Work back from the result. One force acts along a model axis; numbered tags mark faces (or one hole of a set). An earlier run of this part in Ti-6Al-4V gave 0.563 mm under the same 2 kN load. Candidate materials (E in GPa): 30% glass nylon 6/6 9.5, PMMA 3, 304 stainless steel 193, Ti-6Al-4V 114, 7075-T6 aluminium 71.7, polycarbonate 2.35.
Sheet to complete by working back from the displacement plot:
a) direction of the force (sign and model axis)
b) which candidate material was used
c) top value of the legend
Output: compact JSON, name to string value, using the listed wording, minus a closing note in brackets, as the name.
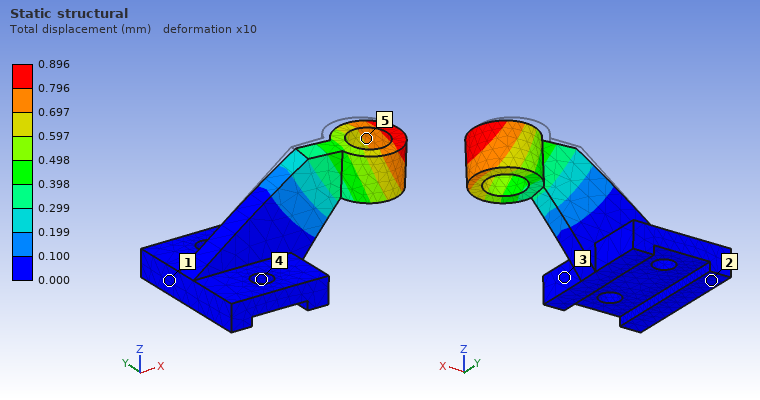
{"direction of the force": "-Y", "which candidate material was used": "7075-T6 aluminium", "top value of the legend": "0.896 mm"}
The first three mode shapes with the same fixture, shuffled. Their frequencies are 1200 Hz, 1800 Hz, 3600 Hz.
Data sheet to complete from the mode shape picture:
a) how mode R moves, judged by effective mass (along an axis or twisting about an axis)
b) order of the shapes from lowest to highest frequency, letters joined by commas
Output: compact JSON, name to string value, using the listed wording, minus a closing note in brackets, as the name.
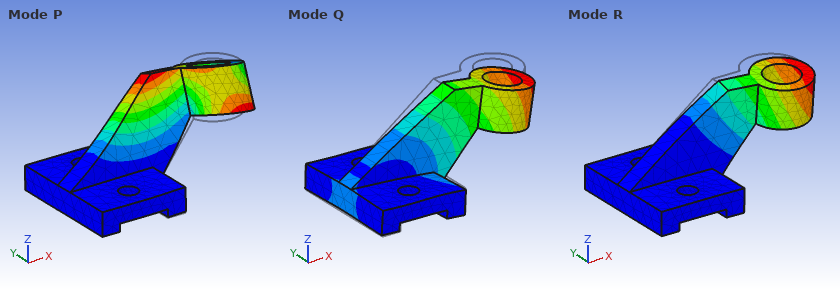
{"how mode R moves, judged by effective mass": "along Y", "order of the shapes from lowest to highest frequency, letters joined by commas": "R, Q, P"}
